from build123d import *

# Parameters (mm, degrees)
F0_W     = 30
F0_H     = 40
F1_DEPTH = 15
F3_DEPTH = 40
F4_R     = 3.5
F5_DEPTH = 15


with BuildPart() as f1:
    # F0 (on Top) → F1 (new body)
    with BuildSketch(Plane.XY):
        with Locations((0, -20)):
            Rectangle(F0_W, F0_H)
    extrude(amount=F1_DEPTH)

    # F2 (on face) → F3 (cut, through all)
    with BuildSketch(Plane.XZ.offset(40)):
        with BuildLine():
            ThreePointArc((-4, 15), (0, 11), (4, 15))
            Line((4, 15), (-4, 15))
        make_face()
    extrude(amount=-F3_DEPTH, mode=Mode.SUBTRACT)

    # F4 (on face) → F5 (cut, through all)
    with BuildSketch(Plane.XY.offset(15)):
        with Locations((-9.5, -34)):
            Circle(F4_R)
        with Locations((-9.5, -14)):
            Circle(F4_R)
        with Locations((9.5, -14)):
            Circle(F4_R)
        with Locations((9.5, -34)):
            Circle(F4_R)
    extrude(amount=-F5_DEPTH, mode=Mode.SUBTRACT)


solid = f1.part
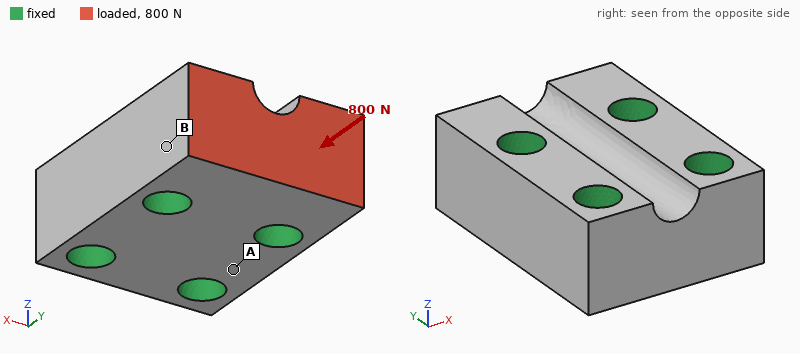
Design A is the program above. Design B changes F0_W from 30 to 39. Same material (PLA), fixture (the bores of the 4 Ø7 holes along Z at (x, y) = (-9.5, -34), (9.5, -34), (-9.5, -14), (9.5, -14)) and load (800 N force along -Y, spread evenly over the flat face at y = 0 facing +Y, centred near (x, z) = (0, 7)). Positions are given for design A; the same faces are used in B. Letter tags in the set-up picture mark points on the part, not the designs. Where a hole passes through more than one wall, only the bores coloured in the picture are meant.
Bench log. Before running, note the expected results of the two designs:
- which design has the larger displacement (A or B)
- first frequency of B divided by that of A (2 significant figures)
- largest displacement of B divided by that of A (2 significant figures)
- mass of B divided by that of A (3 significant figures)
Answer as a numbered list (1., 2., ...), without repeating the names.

1. B
2. 0.94
3. 1.1
4. 1.37
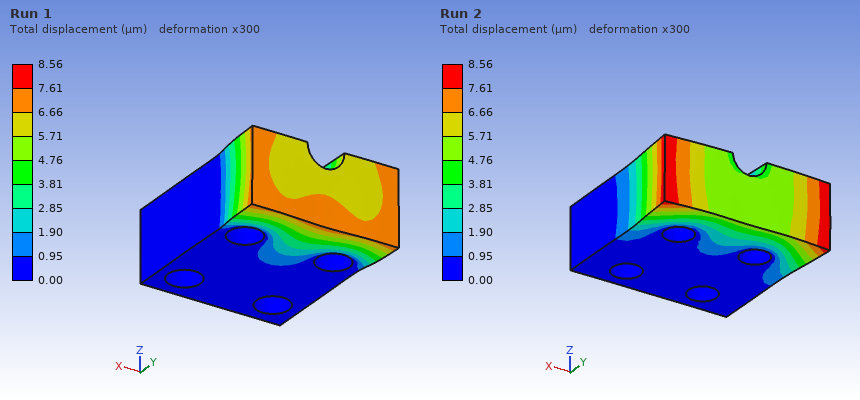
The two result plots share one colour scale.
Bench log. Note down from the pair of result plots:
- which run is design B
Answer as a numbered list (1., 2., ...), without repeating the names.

1. Run 2
